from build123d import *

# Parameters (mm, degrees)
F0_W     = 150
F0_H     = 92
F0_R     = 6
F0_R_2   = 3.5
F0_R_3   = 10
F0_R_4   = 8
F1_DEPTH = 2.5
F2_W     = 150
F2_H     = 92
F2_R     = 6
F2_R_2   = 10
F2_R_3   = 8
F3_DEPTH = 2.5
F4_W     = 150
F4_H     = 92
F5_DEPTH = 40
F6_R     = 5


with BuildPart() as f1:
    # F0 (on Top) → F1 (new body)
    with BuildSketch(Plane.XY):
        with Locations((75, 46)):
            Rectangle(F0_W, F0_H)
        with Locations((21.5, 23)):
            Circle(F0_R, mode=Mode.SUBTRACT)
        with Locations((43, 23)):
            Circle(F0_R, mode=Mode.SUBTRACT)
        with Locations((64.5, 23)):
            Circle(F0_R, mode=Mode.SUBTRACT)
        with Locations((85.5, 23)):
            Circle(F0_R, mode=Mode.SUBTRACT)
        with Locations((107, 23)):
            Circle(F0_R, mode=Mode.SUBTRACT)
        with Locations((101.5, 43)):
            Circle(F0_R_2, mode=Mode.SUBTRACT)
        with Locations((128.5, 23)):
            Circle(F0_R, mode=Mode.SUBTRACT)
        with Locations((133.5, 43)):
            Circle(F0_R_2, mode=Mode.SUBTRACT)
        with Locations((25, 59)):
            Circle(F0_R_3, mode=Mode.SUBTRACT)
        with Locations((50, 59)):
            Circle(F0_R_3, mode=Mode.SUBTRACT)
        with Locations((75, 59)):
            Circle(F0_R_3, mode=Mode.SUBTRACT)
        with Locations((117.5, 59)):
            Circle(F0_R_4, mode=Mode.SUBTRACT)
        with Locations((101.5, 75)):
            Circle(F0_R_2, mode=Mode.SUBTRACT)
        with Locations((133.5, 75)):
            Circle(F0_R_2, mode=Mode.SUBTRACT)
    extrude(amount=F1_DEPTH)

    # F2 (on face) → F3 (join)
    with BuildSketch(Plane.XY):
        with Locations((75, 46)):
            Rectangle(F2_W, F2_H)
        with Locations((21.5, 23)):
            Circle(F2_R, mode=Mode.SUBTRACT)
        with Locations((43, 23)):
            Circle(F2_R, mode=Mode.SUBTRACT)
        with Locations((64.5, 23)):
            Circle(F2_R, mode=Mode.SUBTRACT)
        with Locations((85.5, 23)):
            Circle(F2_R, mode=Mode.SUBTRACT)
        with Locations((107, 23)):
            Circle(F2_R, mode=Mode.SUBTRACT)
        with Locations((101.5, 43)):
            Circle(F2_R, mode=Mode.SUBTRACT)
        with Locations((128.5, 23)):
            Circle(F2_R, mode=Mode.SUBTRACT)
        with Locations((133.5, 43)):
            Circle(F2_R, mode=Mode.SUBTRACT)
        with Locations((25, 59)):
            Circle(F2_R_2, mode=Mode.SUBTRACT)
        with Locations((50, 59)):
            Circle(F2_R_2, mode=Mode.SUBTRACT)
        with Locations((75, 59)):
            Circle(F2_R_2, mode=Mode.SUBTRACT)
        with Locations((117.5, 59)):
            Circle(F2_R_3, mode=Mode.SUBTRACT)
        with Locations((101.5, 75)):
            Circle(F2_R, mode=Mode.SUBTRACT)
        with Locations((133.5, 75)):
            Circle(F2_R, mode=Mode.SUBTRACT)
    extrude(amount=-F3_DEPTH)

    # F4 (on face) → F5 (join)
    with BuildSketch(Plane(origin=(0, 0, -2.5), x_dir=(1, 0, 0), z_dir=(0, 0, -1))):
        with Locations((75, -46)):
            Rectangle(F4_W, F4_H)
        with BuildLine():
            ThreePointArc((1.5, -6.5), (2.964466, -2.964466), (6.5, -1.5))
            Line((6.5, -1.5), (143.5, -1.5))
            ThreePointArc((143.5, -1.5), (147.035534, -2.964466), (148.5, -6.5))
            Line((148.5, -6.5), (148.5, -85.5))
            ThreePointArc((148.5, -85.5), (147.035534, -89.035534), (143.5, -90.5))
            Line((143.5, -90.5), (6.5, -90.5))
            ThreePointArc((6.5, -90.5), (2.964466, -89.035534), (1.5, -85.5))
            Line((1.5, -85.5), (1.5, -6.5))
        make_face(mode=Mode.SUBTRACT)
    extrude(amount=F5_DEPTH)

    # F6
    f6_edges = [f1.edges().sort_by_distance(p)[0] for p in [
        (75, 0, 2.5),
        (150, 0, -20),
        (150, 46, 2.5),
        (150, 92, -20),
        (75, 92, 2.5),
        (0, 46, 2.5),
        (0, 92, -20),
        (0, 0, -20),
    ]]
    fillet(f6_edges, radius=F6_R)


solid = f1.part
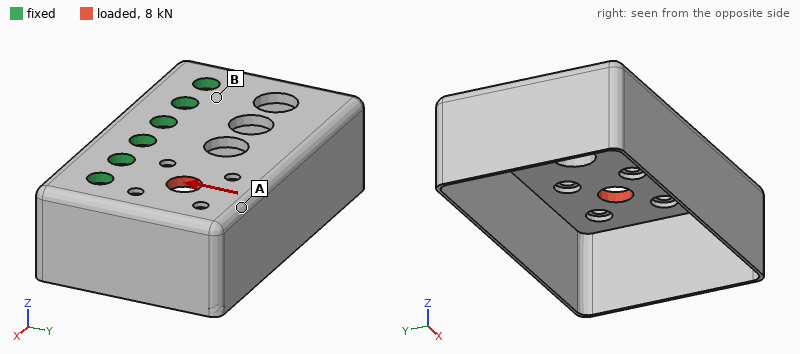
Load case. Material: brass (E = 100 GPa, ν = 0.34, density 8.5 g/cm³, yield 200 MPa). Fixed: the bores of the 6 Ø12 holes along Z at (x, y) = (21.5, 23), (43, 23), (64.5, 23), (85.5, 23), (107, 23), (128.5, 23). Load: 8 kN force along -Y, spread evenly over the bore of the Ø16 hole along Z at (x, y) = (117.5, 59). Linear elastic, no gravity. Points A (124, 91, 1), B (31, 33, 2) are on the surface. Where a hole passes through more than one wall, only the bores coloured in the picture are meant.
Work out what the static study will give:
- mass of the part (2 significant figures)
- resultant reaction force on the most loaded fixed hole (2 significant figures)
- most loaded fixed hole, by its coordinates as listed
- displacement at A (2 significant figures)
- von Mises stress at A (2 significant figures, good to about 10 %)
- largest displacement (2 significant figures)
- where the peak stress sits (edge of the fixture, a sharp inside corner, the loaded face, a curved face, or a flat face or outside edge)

720 g
4.5 kN
(128.5, 23)
17 µm
18 MPa
20 µm
a curved face
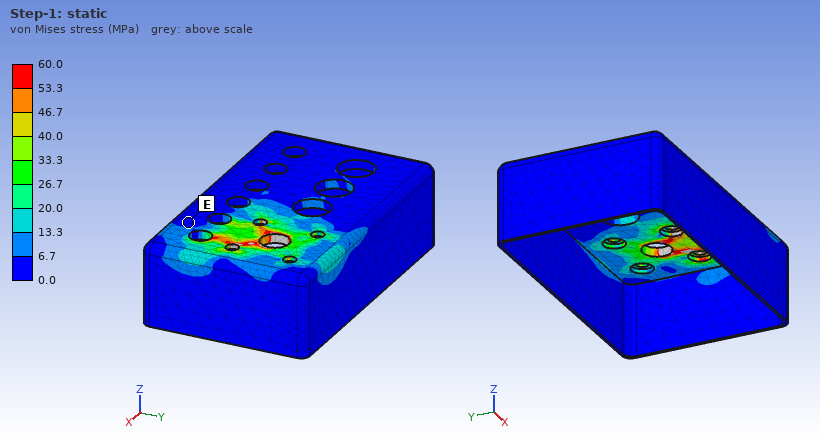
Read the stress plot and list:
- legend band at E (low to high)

0.0 to 6.7 MPa
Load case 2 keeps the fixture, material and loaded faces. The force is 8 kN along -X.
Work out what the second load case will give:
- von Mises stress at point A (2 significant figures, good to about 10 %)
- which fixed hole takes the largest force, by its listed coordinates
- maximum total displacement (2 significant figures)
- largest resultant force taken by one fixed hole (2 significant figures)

13 MPa
(128.5, 23)
33 µm
4.3 kN
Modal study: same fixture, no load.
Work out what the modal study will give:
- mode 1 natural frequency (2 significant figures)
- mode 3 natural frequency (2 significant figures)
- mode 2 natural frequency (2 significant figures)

580 Hz
740 Hz
640 Hz
